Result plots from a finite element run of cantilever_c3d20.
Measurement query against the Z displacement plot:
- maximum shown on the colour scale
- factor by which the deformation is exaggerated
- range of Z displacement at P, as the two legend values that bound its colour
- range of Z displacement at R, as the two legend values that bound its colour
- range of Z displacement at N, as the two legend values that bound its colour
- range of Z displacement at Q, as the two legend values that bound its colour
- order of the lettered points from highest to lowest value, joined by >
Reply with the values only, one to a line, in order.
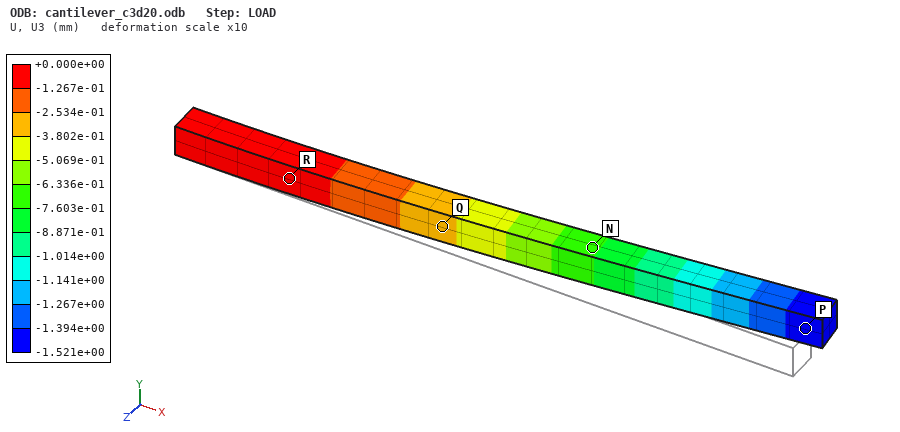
+0.000e+00 mm
10
-1.521e+00 to -1.394e+00 mm
-1.267e-01 to +0.000e+00 mm
-7.603e-01 to -6.336e-01 mm
-3.802e-01 to -2.534e-01 mm
R > Q > N > P
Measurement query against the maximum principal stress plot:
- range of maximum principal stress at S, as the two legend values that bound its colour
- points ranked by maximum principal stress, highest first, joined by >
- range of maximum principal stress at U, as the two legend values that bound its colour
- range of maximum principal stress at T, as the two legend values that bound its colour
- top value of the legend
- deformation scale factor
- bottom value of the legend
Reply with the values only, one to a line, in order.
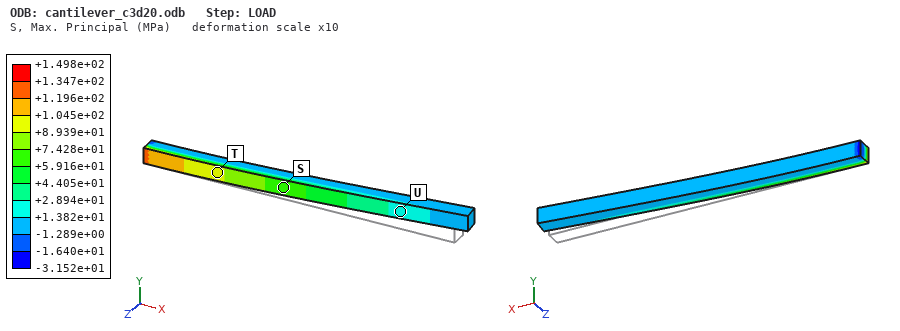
+5.916e+01 to +7.428e+01 MPa
T > S > U
+1.382e+01 to +2.894e+01 MPa
+8.939e+01 to +1.045e+02 MPa
+1.498e+02 MPa
10
-3.152e+01 MPa
